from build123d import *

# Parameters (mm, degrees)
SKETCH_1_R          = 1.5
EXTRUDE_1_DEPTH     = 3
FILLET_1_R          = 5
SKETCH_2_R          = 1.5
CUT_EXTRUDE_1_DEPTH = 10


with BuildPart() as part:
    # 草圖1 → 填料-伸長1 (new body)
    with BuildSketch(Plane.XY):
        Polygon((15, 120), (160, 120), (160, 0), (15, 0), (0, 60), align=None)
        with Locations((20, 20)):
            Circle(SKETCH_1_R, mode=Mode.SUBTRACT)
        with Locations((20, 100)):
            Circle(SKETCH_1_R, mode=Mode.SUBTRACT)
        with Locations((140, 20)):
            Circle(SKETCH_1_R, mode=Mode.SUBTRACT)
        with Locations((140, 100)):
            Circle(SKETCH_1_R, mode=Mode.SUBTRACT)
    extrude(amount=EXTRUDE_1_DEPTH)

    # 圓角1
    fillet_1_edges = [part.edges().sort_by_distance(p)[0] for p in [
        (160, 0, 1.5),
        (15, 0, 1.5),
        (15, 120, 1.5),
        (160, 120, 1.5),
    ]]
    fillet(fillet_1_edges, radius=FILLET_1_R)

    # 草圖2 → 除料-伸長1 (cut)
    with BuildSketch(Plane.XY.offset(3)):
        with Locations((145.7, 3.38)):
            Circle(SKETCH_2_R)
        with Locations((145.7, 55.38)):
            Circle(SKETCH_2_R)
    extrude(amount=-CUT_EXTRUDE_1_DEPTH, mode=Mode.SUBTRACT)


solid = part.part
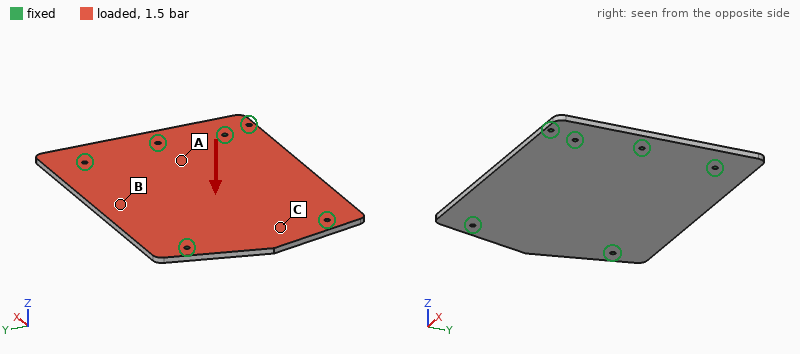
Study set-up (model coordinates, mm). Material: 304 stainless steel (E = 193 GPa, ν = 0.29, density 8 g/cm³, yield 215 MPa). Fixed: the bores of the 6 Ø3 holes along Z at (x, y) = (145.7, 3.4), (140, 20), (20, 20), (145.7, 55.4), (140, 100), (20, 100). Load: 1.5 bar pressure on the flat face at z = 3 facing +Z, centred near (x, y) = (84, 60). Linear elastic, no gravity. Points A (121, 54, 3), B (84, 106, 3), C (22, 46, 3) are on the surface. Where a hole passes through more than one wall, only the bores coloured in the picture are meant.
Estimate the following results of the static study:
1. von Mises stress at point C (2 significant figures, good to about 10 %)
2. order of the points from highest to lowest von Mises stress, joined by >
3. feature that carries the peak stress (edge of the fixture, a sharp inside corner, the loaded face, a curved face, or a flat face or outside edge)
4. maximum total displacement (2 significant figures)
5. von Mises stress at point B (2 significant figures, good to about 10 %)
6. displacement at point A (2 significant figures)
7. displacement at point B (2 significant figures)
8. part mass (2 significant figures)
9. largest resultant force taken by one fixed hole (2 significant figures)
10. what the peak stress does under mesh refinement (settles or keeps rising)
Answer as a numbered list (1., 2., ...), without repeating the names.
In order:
1. 39 MPa
2. B > C > A
3. edge of the fixture
4. 0.27 mm
5. 69 MPa
6. 0.11 mm
7. 0.25 mm
8. 440 g
9. 640 N
10. keeps rising
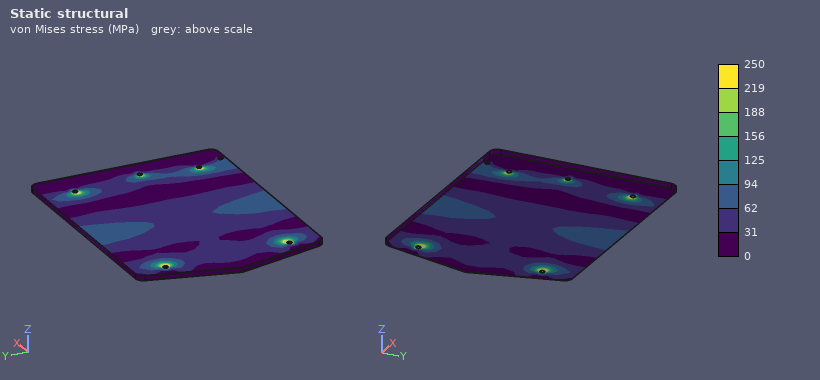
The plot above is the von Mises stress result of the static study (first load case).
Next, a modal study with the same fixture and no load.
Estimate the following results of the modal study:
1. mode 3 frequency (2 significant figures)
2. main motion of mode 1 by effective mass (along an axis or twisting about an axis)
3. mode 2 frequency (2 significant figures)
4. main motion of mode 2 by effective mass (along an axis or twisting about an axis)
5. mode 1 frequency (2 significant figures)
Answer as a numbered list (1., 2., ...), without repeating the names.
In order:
1. 1700 Hz
2. along Z
3. 1100 Hz
4. twisting about X
5. 880 Hz
